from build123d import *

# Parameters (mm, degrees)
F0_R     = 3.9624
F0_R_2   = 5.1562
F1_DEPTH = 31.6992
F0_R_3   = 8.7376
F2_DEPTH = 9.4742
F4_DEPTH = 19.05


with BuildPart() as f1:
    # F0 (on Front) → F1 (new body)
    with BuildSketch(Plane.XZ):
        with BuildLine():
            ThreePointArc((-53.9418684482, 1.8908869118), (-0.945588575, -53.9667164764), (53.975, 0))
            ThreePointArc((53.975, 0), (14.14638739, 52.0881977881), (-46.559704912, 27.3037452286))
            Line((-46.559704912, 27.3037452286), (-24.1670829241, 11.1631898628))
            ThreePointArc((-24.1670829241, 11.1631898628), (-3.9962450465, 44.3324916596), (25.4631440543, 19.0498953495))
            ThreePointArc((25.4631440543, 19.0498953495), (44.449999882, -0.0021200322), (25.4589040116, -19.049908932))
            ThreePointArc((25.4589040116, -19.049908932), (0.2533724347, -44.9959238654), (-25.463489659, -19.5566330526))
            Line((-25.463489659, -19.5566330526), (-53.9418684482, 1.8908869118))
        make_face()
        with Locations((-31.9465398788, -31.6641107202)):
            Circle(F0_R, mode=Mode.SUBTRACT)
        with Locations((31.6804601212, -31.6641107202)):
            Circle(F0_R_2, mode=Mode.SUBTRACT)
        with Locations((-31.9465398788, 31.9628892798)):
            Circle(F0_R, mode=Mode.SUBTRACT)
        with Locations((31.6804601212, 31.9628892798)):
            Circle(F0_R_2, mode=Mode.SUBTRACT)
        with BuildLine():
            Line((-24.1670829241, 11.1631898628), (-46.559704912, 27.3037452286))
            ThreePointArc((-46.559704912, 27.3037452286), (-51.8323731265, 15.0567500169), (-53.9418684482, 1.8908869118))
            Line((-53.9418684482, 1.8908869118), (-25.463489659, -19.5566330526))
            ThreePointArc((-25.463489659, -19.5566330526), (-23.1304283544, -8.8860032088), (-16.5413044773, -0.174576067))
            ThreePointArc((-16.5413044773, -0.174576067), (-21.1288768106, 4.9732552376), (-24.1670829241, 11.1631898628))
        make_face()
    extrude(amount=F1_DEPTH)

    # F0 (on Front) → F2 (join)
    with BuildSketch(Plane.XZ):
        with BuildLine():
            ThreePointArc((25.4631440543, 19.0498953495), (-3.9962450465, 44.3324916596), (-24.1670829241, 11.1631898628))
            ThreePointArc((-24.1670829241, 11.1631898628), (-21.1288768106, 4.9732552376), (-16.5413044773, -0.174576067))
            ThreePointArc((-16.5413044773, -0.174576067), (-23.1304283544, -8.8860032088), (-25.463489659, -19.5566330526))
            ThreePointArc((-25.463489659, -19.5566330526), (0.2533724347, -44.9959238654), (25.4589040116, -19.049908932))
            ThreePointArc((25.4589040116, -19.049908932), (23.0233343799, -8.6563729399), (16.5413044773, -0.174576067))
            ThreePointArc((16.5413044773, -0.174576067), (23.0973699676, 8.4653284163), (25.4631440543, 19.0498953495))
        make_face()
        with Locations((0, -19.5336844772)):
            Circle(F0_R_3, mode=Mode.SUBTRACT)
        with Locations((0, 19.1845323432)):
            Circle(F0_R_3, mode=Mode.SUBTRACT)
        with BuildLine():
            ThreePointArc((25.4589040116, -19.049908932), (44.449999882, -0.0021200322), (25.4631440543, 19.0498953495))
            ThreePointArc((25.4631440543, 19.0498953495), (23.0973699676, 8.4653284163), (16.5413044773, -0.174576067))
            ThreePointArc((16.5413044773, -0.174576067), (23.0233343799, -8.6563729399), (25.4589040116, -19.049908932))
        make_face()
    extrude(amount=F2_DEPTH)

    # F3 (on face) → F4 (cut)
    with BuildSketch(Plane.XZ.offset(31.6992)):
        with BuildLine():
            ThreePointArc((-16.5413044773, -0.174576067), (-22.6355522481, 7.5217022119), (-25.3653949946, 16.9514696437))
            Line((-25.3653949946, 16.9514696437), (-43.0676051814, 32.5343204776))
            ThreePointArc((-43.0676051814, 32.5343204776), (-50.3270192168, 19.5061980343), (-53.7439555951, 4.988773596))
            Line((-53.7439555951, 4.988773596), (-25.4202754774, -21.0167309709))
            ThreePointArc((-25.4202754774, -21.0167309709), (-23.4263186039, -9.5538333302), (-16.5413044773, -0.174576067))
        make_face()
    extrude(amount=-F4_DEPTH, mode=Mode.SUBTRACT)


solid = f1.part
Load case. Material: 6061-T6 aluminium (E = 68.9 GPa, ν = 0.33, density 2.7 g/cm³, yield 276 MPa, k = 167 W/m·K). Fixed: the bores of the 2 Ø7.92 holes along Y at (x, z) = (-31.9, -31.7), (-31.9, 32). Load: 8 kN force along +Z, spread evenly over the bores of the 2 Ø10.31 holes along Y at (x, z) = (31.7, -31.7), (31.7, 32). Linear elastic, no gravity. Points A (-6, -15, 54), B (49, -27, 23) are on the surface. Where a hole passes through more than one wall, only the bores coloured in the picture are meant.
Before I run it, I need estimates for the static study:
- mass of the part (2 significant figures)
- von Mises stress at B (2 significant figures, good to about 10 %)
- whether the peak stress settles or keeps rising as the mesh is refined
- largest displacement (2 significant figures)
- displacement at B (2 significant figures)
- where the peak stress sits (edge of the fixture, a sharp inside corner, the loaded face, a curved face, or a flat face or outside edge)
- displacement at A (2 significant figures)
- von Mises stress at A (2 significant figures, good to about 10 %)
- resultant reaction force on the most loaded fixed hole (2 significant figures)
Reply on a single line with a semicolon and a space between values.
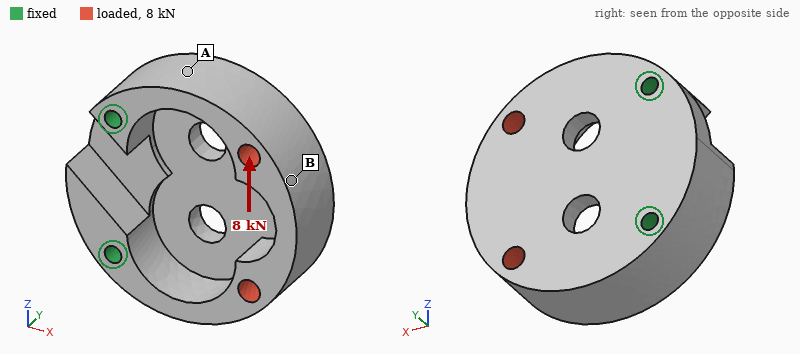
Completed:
430 g; 9.3 MPa; keeps rising; 93 µm; 83 µm; edge of the fixture; 34 µm; 19 MPa; 7.9 kN
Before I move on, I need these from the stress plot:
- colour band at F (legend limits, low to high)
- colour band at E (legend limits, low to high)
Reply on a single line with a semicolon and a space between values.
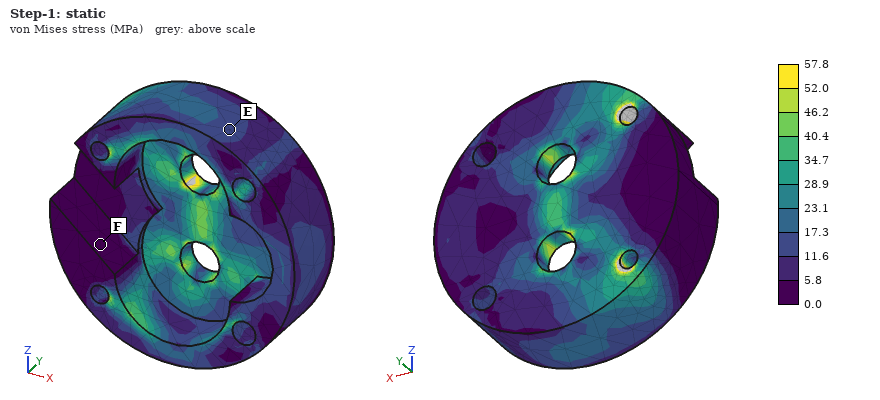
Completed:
0.0 to 5.8 MPa; 11.6 to 17.3 MPa
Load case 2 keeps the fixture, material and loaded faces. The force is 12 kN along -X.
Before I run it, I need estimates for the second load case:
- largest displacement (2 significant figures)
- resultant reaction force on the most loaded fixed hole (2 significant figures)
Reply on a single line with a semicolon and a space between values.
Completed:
0.11 mm; 6.1 kN
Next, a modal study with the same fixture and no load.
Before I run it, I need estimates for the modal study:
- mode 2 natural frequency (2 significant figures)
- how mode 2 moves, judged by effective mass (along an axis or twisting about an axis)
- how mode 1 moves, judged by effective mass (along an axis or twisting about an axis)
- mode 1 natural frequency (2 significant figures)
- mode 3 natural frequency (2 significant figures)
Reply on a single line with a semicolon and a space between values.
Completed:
3800 Hz; along Z; along Y; 2000 Hz; 5700 Hz
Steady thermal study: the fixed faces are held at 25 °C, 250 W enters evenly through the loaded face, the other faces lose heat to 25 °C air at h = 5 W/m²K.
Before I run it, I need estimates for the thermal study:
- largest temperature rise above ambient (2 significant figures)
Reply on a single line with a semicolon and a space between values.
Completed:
84 K
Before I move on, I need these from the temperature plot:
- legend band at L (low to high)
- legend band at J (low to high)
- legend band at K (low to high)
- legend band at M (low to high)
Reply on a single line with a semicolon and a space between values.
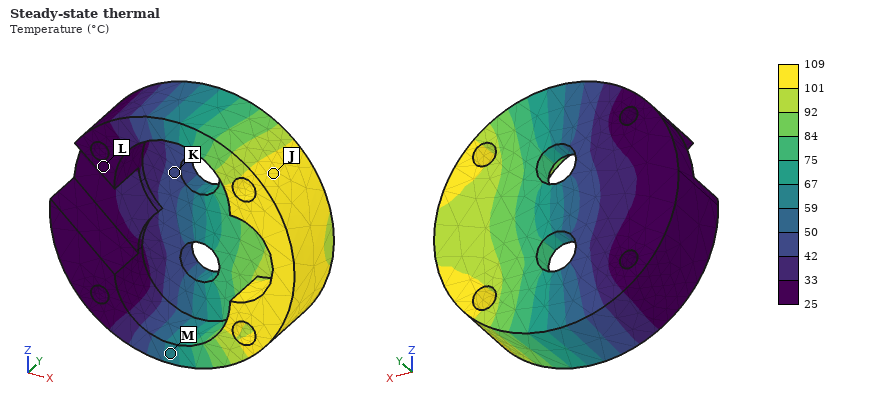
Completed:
25 to 33 °C; 101 to 109 °C; 42 to 50 °C; 59 to 67 °C
